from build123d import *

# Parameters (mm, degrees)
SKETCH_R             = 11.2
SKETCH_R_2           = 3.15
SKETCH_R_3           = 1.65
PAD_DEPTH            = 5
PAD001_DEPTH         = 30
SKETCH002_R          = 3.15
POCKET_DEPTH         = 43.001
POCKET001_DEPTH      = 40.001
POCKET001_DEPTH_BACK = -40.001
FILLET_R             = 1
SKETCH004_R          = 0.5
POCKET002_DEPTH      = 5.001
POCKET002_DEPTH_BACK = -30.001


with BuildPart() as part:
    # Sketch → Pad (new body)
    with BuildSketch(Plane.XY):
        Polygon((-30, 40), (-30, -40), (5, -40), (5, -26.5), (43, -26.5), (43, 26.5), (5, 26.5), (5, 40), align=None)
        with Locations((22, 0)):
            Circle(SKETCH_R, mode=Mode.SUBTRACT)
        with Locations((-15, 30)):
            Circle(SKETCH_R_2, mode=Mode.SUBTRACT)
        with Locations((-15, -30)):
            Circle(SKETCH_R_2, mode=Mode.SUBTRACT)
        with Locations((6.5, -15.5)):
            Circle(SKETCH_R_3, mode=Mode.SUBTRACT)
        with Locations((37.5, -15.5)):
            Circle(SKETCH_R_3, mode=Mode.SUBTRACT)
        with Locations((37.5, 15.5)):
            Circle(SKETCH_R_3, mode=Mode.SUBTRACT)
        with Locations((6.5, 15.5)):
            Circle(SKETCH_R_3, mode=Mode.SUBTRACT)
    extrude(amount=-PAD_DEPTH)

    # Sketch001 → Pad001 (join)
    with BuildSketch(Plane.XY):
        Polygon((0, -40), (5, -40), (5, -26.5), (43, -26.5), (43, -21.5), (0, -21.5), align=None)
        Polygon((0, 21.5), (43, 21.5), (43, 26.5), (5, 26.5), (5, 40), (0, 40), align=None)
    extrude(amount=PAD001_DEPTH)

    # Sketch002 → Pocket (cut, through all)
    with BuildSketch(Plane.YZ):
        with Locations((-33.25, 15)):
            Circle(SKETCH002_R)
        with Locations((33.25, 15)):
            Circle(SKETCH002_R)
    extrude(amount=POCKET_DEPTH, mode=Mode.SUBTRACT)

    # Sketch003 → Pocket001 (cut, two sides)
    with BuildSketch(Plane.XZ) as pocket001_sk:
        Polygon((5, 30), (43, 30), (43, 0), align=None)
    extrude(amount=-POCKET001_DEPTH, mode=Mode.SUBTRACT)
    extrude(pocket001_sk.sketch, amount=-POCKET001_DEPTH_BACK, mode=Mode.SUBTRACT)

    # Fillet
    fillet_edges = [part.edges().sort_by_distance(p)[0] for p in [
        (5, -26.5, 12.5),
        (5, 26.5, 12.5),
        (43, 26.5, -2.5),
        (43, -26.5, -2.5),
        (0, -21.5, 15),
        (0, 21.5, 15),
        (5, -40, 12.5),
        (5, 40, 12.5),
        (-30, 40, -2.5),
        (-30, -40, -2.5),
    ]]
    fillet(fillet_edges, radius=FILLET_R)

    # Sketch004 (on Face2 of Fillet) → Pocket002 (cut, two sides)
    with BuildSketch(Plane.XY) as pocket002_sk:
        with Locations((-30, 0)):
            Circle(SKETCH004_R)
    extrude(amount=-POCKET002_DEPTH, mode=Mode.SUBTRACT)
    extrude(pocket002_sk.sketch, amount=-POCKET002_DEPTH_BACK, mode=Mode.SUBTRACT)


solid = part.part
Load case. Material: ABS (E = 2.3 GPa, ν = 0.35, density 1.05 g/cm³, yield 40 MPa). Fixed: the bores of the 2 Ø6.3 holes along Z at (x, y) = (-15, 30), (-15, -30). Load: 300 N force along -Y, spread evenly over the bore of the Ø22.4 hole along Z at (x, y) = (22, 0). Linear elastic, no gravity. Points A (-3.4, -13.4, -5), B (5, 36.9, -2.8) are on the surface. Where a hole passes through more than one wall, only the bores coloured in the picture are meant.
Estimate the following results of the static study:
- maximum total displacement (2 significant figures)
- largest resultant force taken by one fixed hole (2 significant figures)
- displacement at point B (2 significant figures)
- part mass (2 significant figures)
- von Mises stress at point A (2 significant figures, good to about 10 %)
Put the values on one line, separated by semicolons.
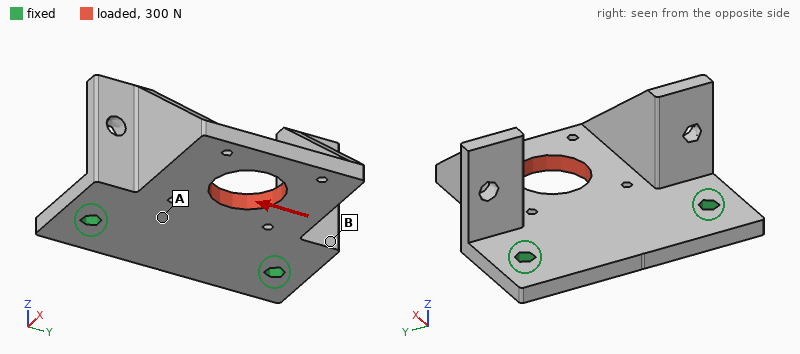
0.13 mm; 230 N; 0.027 mm; 34 g; 1.5 MPa
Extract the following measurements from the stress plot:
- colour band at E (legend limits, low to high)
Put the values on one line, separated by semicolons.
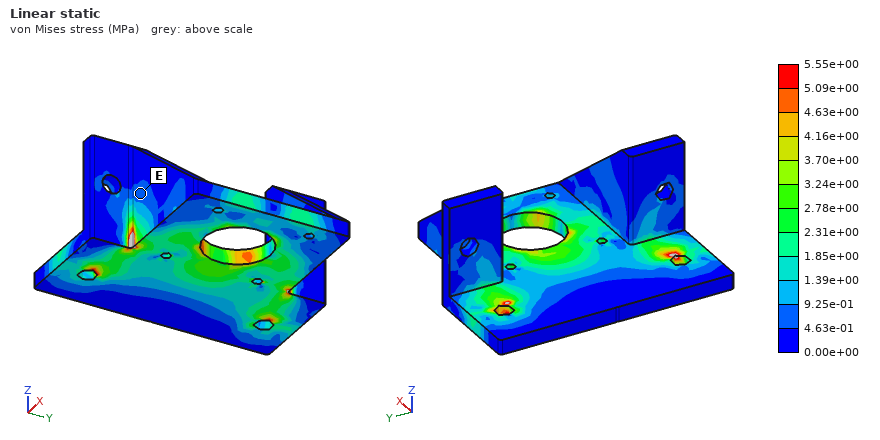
4.63e-01 to 9.25e-01 MPa
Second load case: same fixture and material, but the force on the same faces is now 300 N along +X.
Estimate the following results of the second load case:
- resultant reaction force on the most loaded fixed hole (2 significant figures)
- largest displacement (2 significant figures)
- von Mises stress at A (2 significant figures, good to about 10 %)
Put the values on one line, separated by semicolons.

160 N; 59 µm; 1.0 MPa
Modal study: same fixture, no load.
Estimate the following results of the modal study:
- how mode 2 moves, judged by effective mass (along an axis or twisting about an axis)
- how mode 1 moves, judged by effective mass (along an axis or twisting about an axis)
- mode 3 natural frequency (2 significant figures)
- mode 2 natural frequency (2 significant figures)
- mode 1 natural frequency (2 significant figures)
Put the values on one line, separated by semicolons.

twisting about X; along Z; 1000 Hz; 700 Hz; 350 Hz
